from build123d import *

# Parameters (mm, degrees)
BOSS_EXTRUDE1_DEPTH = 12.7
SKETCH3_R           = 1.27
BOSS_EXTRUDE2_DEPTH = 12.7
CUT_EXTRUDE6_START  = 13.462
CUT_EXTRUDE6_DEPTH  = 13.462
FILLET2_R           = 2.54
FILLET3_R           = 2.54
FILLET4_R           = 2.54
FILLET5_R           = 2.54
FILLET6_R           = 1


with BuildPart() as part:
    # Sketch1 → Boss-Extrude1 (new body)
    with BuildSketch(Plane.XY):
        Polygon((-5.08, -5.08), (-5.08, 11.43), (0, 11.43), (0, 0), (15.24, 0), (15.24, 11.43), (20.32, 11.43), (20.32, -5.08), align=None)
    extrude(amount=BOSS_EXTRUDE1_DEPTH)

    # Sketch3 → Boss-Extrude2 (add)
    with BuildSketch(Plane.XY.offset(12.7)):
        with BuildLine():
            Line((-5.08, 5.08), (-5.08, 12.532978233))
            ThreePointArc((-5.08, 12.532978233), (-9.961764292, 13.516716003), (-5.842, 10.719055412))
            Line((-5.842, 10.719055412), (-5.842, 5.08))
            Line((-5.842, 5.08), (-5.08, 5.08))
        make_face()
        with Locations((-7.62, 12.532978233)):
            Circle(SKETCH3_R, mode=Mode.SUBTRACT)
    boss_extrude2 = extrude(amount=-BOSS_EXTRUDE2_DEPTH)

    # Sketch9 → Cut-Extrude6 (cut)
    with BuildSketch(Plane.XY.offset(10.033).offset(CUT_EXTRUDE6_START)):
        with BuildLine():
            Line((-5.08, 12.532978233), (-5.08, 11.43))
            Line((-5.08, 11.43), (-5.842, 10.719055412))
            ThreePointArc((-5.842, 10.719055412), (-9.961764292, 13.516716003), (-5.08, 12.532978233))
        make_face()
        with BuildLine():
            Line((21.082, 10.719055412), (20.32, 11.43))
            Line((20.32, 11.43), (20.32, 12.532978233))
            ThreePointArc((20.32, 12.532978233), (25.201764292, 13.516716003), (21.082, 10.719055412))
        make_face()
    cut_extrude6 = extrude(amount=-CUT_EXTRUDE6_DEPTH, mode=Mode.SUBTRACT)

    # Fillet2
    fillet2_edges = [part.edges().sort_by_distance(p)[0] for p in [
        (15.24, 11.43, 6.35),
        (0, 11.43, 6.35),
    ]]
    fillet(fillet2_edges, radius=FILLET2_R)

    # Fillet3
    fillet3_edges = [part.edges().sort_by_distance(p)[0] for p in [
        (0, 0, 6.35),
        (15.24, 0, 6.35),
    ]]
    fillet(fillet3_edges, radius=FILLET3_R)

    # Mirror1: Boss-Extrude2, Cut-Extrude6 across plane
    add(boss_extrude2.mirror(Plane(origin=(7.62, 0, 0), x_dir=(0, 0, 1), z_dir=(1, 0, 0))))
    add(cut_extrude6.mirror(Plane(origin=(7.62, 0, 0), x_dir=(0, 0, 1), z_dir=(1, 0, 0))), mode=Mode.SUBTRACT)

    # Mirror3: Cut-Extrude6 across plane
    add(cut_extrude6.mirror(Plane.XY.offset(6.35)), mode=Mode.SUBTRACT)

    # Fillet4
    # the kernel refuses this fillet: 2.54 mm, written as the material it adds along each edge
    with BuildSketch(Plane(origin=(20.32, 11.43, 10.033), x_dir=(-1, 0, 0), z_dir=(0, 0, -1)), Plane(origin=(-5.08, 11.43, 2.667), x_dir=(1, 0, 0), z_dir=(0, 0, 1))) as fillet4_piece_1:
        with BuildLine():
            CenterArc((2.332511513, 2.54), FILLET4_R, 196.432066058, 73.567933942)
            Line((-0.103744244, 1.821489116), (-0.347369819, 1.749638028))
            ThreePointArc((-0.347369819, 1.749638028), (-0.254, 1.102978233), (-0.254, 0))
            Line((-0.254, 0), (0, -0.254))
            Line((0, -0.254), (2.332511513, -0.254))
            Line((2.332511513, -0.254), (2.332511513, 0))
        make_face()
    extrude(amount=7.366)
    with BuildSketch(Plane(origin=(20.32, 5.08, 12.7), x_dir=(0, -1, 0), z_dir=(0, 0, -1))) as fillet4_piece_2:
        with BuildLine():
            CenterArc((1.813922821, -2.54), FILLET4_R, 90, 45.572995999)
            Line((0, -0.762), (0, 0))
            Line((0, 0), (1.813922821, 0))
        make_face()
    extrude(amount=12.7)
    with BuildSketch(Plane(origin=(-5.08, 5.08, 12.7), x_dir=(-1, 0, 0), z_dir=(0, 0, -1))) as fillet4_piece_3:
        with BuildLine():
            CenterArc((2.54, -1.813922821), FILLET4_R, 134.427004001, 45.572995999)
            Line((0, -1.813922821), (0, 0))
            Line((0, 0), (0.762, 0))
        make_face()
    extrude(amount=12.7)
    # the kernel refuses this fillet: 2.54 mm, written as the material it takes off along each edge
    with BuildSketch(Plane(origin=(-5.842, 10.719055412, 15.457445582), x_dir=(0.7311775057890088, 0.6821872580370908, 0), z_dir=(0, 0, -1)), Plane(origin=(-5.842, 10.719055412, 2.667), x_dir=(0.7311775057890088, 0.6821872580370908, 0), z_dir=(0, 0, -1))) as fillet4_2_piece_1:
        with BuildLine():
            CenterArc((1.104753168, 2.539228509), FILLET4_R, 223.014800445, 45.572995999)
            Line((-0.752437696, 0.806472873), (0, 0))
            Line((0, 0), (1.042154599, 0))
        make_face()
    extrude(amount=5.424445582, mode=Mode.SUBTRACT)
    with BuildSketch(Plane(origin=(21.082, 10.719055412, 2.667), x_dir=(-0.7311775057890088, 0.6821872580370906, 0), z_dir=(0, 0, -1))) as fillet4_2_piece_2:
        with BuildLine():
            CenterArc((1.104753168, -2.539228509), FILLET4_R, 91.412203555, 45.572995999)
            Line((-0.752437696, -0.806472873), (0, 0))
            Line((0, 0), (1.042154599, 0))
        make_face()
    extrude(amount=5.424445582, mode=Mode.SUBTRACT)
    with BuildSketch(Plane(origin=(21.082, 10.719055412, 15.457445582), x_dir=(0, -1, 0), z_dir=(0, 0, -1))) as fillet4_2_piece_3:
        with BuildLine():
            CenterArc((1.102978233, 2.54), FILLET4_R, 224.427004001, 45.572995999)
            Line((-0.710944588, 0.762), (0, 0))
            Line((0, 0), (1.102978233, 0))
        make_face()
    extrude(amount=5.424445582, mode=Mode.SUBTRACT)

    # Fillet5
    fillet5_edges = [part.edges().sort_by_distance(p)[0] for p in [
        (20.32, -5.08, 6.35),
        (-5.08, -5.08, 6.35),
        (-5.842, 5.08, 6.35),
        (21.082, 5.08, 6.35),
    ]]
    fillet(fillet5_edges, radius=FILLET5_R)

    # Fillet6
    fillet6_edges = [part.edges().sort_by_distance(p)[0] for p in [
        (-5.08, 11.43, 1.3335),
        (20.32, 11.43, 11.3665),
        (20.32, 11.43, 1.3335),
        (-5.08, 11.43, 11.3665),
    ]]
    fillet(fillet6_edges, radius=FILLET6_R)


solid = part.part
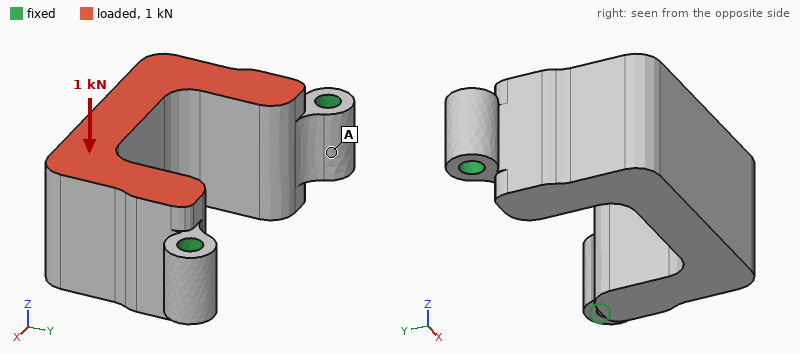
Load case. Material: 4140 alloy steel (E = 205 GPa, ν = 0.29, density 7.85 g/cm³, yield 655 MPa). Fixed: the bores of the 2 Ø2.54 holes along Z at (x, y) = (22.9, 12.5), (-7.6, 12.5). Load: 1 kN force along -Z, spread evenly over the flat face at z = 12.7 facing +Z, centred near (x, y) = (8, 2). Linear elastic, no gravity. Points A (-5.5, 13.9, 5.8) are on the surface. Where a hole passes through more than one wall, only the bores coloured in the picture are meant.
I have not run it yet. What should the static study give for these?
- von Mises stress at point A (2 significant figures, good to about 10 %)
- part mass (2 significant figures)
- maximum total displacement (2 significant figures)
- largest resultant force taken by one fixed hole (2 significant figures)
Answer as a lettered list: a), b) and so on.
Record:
a) 53 MPa
b) 27 g
c) 31 µm
d) 500 N
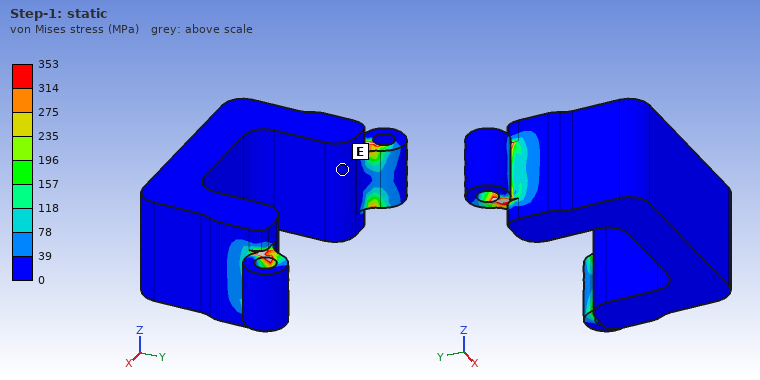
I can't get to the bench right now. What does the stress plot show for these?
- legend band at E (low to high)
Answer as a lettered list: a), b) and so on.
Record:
a) 0 to 39 MPa
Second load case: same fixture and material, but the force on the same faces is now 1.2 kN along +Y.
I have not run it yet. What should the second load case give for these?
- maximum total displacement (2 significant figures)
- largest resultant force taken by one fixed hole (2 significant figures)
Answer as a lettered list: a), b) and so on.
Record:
a) 25 µm
b) 630 N
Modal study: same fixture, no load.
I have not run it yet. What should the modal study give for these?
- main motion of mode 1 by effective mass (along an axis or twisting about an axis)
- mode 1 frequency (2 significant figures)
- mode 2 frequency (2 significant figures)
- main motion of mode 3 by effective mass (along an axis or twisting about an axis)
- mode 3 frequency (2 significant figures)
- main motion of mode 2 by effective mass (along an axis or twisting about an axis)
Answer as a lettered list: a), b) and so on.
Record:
a) along Z
b) 6500 Hz
c) 12 kHz
d) twisting about Y
e) 15 kHz
f) along X
